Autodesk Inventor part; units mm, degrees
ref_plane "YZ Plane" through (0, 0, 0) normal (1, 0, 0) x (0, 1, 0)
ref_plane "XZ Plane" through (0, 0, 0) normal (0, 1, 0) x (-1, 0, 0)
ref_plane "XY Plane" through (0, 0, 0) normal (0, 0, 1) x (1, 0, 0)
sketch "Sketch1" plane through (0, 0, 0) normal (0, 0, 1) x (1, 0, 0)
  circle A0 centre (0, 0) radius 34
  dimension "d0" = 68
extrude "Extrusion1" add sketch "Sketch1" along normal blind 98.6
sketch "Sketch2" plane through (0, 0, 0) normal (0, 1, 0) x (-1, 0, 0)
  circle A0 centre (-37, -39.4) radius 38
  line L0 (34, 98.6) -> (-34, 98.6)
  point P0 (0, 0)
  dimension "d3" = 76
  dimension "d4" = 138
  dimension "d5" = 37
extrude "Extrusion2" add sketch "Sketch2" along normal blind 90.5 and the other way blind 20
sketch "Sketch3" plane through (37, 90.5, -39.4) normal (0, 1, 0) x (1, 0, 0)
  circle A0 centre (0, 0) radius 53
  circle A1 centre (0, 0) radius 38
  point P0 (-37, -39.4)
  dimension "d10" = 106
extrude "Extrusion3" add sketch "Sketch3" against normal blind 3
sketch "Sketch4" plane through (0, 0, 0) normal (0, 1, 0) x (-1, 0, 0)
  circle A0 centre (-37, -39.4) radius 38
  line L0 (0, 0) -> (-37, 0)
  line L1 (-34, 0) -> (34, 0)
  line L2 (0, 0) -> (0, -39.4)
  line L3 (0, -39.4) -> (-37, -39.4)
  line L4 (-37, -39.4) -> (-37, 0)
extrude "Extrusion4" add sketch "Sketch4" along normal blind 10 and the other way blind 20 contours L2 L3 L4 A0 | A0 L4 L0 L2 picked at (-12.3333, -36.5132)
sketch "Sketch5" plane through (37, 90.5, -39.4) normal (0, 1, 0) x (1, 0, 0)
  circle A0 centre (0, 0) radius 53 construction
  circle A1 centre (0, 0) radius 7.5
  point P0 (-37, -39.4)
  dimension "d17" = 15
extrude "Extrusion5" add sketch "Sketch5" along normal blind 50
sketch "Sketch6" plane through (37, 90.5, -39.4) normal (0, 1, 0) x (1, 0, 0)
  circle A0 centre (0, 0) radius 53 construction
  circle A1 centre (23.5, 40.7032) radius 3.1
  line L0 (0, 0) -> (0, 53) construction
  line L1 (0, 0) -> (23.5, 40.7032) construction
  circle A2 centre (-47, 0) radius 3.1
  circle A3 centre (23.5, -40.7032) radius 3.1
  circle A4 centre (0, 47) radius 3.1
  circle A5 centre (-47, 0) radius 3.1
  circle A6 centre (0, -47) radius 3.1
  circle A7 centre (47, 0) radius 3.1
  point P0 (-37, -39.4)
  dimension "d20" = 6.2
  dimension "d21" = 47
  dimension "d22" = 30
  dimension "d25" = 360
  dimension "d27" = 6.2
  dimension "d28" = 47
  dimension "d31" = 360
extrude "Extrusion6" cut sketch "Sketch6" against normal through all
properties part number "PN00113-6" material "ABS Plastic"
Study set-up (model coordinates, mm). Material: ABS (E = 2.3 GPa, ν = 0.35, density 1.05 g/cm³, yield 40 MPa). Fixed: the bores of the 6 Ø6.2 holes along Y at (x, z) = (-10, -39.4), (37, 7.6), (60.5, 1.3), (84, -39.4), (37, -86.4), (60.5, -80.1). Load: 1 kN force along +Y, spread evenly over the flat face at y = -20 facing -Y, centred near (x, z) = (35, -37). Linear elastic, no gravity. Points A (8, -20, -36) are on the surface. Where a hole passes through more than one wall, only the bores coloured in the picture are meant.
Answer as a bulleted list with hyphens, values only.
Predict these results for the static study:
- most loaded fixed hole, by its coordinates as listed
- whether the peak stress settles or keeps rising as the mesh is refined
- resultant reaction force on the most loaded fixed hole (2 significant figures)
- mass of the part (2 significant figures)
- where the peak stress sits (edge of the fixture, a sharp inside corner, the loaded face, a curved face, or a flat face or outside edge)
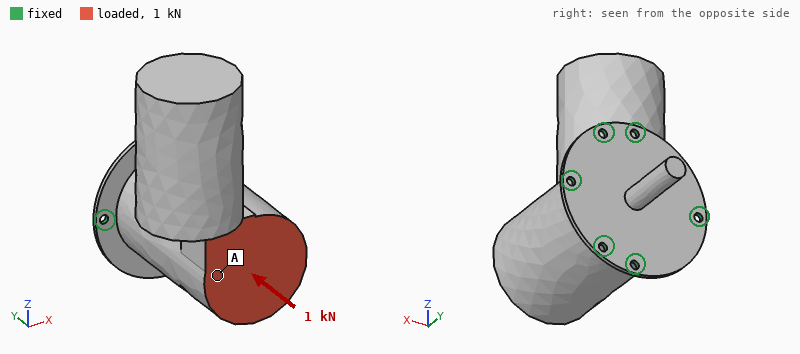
- (-10, -39.4)
- keeps rising
- 300 N
- 930 g
- edge of the fixture
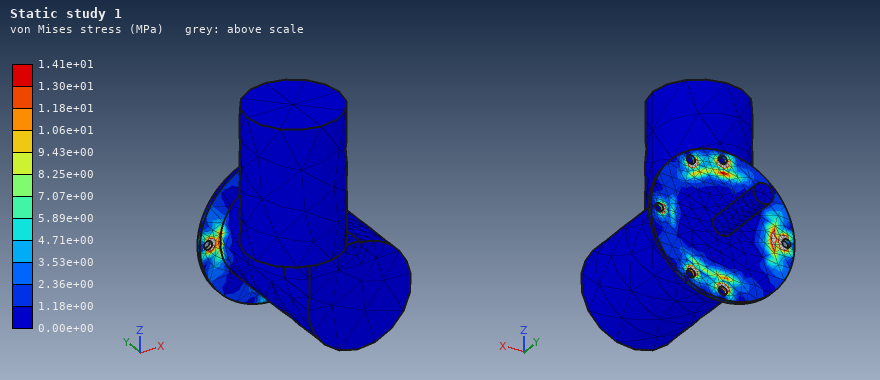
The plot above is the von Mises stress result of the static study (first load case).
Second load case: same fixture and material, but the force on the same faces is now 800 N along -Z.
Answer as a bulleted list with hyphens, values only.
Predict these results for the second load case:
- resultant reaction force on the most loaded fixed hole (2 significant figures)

- 650 N
